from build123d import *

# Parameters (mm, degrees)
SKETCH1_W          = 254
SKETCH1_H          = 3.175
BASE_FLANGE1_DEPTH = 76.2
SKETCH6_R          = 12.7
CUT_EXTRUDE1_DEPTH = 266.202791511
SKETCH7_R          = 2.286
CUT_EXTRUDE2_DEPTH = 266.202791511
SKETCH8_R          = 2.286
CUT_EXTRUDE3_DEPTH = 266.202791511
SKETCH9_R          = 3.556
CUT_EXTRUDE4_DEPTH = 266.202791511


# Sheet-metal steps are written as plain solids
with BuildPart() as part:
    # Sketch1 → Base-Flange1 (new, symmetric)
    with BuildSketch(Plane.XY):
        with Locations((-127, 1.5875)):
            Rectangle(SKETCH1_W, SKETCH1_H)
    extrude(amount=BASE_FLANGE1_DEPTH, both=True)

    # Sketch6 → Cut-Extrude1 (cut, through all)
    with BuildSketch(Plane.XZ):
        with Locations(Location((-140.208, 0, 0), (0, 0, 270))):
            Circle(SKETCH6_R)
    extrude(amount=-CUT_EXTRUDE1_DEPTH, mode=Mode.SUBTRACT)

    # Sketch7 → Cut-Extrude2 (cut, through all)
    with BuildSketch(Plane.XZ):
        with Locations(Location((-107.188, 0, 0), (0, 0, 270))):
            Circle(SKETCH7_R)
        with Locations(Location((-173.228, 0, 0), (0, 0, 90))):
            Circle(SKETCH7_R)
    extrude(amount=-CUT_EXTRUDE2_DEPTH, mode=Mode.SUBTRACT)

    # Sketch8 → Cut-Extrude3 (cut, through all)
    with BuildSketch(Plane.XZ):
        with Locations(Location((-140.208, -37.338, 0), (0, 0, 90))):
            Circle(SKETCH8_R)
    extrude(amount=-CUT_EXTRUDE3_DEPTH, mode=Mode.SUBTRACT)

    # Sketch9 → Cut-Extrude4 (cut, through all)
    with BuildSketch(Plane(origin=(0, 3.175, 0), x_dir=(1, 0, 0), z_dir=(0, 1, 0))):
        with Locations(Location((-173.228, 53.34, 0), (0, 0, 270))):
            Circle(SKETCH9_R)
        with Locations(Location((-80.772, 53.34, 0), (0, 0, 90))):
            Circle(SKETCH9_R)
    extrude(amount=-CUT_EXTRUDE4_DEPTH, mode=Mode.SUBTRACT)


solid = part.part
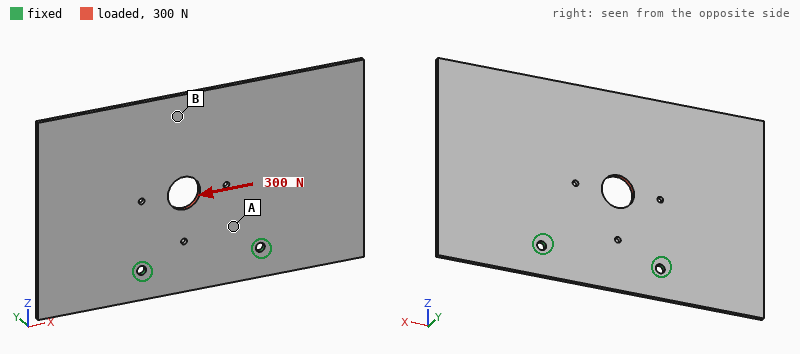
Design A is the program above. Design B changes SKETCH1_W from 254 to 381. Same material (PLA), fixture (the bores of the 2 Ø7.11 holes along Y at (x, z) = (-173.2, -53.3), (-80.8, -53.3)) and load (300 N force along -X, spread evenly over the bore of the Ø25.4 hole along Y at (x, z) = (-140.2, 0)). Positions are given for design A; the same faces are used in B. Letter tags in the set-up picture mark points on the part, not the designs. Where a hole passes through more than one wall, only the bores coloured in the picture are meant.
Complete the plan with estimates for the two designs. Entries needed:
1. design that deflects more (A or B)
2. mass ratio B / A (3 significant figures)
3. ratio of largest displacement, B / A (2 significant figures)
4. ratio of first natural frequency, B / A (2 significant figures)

B
1.51
1.3
0.66
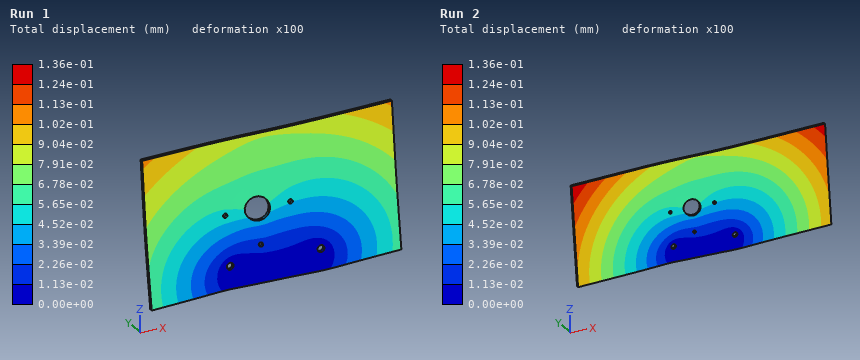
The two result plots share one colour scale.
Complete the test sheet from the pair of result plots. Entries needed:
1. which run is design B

Run 2
